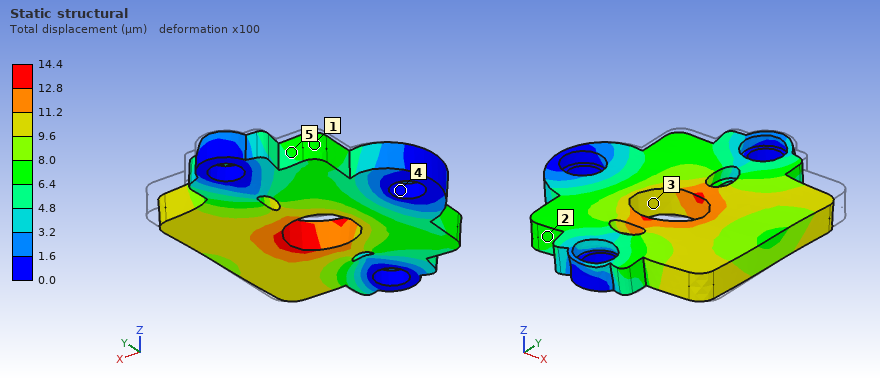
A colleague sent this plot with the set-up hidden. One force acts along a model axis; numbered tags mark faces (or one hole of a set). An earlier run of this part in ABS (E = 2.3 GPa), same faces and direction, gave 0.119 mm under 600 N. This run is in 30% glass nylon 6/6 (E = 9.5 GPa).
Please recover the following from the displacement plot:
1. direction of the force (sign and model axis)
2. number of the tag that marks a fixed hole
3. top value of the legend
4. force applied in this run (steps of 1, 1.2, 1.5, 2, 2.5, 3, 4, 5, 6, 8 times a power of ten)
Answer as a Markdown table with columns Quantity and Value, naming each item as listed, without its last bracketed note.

| Quantity | Value |
|---|---|
| direction of the force | -Y |
| number of the tag that marks a fixed hole | 4 |
| top value of the legend | 14.4 µm |
| force applied in this run | 300 N |
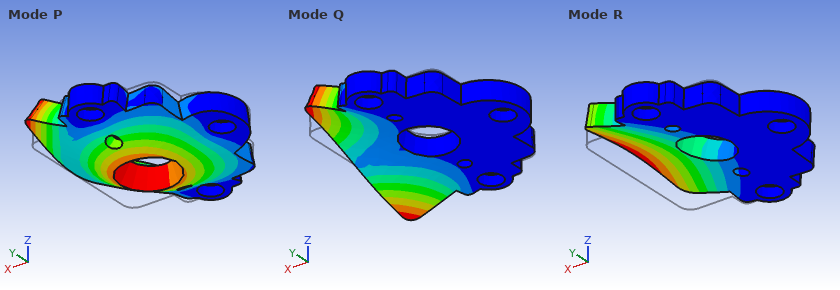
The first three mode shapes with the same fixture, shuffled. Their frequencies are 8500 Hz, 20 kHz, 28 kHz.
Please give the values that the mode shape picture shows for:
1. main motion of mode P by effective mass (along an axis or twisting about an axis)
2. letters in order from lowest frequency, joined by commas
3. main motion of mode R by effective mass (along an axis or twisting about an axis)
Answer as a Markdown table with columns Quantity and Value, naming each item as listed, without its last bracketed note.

| Quantity | Value |
|---|---|
| main motion of mode P by effective mass | along Z |
| letters in order from lowest frequency, joined by commas | R, Q, P |
| main motion of mode R by effective mass | along Z |
